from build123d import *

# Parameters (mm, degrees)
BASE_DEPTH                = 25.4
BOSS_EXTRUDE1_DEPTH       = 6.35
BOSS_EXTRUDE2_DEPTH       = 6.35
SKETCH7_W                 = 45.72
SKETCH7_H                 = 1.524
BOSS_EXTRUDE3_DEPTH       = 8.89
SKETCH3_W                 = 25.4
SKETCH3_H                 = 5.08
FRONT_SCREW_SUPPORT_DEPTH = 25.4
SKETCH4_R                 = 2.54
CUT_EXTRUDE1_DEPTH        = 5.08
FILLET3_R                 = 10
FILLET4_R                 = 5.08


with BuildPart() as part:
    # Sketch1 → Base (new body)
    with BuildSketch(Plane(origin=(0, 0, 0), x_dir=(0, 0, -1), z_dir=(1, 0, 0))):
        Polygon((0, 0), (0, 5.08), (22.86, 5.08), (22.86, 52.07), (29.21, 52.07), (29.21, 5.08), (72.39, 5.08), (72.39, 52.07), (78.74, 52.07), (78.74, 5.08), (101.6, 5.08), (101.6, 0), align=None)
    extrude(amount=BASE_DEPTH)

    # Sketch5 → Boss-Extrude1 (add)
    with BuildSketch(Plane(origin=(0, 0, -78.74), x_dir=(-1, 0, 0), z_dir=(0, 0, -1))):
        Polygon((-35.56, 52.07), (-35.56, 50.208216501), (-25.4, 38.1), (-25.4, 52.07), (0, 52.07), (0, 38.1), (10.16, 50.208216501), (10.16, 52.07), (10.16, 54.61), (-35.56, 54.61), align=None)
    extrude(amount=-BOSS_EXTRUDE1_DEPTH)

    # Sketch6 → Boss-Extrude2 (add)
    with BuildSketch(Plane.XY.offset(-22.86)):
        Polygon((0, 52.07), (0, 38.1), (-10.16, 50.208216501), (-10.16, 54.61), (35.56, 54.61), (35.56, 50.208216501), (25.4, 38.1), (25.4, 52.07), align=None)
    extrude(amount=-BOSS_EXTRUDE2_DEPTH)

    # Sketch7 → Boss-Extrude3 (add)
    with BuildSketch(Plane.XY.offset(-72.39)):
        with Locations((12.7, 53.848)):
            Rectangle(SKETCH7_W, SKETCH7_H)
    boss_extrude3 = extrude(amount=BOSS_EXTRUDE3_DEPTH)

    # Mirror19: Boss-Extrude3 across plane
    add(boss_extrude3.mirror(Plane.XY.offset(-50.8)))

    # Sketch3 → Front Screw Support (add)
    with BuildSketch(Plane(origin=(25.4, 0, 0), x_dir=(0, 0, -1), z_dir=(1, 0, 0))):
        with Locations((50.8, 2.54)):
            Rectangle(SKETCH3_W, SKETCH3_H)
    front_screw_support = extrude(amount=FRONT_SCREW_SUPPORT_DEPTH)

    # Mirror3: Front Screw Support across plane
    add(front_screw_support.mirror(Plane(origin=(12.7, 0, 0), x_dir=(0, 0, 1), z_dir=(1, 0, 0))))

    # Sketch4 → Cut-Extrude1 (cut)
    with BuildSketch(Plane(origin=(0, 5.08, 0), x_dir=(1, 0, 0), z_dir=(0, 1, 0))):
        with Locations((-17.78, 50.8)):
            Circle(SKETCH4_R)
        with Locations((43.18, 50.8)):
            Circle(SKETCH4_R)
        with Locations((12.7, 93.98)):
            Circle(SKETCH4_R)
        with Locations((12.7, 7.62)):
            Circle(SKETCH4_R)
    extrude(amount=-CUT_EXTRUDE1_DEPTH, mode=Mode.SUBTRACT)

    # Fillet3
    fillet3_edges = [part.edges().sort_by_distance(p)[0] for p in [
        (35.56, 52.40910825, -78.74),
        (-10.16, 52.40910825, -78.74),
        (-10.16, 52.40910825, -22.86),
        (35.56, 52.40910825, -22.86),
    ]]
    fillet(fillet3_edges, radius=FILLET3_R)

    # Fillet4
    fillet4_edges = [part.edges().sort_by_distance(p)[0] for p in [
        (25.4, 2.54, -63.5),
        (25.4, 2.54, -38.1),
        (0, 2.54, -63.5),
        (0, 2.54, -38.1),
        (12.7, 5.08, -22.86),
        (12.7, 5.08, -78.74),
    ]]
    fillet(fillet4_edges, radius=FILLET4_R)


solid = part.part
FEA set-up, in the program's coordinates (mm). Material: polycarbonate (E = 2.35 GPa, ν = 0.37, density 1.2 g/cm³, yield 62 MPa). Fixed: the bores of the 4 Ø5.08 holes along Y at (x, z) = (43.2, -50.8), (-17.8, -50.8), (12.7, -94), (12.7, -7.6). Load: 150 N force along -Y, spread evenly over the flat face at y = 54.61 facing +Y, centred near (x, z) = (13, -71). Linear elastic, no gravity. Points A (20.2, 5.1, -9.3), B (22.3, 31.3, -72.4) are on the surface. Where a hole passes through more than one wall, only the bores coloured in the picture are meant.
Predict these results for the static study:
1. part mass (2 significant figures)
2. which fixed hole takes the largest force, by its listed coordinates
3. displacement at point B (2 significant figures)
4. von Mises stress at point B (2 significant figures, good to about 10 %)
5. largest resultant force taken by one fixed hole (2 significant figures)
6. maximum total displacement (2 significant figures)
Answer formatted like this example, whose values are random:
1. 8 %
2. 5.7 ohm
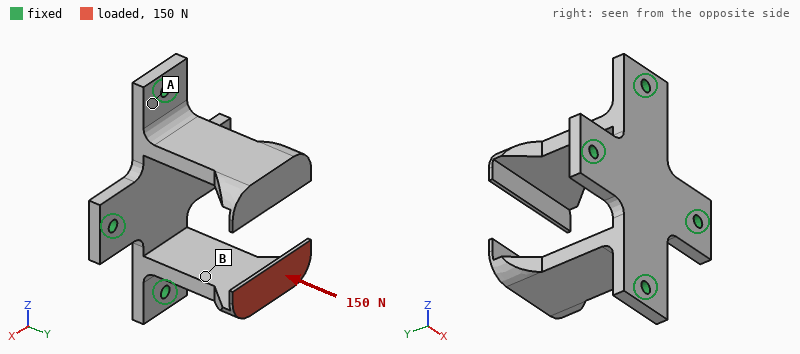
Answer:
1. 47 g
2. (12.7, -94)
3. 0.44 mm
4. 5.3 MPa
5. 79 N
6. 1.4 mm
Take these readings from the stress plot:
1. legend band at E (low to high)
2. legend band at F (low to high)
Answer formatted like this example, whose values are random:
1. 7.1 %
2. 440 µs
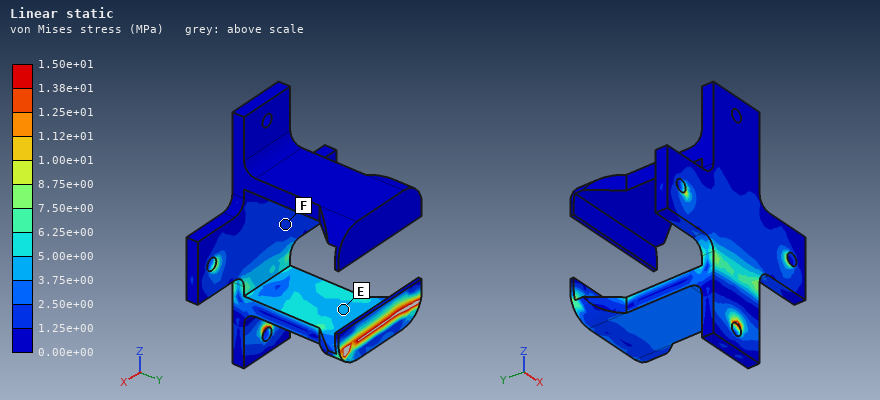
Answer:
1. 3.75e+00 to 5.00e+00 MPa
2. 1.25e+00 to 2.50e+00 MPa
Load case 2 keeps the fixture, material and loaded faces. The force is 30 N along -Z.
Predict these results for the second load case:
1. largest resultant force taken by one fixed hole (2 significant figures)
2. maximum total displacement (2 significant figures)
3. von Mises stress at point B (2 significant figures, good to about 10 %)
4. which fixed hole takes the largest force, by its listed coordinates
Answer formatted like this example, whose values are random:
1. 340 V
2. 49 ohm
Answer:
1. 48 N
2. 1.3 mm
3. 4.2 MPa
4. (12.7, -94)
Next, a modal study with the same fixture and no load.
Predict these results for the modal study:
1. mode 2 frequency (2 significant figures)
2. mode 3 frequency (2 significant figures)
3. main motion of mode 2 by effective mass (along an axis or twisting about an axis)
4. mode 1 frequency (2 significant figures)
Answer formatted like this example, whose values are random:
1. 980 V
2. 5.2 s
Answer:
1. 390 Hz
2. 510 Hz
3. along Z
4. 380 Hz
